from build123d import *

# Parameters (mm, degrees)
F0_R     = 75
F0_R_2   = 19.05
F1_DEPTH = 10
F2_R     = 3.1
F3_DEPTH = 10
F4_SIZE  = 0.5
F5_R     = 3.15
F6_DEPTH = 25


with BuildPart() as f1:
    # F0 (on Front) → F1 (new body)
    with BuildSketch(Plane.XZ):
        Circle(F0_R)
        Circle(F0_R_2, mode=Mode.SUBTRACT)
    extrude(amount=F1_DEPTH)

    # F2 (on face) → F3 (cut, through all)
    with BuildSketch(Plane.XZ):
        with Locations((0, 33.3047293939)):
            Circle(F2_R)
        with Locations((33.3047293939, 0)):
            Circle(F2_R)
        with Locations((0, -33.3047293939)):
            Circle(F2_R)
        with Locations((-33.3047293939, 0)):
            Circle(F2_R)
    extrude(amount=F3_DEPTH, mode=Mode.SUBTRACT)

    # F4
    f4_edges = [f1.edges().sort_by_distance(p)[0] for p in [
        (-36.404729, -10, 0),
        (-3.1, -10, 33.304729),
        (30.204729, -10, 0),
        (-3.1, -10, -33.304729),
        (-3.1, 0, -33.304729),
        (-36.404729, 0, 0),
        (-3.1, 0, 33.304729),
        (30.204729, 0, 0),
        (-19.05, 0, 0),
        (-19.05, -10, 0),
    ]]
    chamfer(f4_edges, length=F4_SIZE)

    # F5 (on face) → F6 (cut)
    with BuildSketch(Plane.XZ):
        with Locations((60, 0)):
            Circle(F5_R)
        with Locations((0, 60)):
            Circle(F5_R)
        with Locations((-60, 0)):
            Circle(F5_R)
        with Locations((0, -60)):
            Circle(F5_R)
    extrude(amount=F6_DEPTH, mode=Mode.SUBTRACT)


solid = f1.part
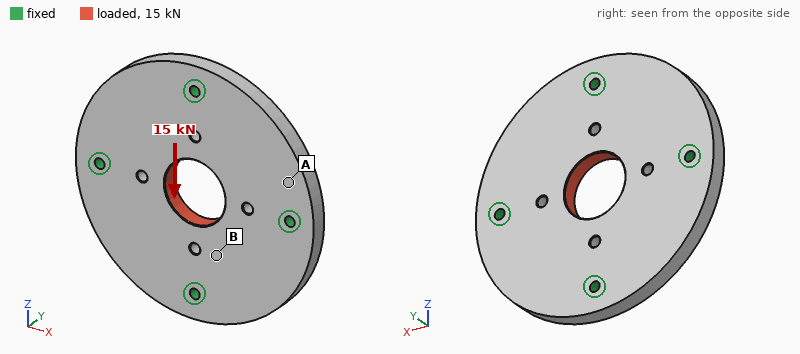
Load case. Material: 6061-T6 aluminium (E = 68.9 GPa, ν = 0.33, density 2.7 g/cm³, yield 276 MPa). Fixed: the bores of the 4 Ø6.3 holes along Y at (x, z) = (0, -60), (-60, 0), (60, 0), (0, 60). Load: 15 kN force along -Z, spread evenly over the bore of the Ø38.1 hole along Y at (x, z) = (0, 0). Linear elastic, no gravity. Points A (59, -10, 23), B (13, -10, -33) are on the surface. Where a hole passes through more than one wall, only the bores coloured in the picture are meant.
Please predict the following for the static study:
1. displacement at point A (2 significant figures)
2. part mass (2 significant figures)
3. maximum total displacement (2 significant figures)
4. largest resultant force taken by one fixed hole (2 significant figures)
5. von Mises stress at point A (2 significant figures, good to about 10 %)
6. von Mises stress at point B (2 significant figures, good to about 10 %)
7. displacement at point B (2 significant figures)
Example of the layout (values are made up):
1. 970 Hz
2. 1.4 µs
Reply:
1. 3.0 µm
2. 440 g
3. 12 µm
4. 4.6 kN
5. 5.2 MPa
6. 11 MPa
7. 7.4 µm
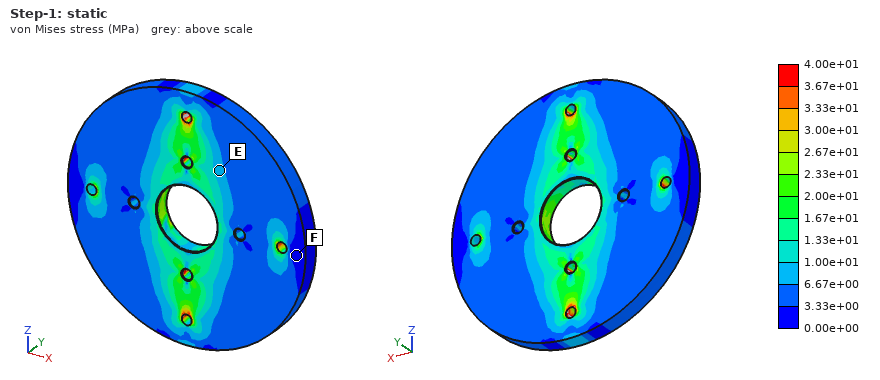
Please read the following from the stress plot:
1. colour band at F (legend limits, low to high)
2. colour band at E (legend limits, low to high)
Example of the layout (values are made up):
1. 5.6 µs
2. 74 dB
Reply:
1. 0.00e+00 to 3.33e+00 MPa
2. 6.67e+00 to 1.00e+01 MPa
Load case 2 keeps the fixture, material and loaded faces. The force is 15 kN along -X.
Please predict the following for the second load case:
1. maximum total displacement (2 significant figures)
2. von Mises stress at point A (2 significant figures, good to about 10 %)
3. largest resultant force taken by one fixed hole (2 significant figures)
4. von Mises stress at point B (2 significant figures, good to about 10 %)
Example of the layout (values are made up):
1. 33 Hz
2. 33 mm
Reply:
1. 12 µm
2. 4.4 MPa
3. 4.6 kN
4. 5.6 MPa
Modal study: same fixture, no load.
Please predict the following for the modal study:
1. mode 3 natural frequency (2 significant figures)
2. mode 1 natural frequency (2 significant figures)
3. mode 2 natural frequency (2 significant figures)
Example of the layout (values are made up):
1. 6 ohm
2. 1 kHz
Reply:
1. 4900 Hz
2. 4400 Hz
3. 4900 Hz
